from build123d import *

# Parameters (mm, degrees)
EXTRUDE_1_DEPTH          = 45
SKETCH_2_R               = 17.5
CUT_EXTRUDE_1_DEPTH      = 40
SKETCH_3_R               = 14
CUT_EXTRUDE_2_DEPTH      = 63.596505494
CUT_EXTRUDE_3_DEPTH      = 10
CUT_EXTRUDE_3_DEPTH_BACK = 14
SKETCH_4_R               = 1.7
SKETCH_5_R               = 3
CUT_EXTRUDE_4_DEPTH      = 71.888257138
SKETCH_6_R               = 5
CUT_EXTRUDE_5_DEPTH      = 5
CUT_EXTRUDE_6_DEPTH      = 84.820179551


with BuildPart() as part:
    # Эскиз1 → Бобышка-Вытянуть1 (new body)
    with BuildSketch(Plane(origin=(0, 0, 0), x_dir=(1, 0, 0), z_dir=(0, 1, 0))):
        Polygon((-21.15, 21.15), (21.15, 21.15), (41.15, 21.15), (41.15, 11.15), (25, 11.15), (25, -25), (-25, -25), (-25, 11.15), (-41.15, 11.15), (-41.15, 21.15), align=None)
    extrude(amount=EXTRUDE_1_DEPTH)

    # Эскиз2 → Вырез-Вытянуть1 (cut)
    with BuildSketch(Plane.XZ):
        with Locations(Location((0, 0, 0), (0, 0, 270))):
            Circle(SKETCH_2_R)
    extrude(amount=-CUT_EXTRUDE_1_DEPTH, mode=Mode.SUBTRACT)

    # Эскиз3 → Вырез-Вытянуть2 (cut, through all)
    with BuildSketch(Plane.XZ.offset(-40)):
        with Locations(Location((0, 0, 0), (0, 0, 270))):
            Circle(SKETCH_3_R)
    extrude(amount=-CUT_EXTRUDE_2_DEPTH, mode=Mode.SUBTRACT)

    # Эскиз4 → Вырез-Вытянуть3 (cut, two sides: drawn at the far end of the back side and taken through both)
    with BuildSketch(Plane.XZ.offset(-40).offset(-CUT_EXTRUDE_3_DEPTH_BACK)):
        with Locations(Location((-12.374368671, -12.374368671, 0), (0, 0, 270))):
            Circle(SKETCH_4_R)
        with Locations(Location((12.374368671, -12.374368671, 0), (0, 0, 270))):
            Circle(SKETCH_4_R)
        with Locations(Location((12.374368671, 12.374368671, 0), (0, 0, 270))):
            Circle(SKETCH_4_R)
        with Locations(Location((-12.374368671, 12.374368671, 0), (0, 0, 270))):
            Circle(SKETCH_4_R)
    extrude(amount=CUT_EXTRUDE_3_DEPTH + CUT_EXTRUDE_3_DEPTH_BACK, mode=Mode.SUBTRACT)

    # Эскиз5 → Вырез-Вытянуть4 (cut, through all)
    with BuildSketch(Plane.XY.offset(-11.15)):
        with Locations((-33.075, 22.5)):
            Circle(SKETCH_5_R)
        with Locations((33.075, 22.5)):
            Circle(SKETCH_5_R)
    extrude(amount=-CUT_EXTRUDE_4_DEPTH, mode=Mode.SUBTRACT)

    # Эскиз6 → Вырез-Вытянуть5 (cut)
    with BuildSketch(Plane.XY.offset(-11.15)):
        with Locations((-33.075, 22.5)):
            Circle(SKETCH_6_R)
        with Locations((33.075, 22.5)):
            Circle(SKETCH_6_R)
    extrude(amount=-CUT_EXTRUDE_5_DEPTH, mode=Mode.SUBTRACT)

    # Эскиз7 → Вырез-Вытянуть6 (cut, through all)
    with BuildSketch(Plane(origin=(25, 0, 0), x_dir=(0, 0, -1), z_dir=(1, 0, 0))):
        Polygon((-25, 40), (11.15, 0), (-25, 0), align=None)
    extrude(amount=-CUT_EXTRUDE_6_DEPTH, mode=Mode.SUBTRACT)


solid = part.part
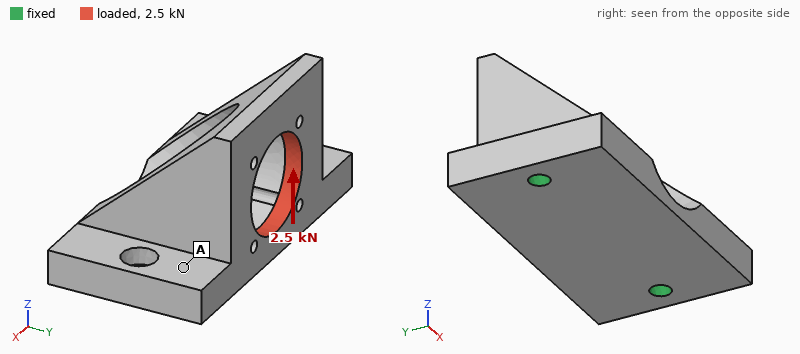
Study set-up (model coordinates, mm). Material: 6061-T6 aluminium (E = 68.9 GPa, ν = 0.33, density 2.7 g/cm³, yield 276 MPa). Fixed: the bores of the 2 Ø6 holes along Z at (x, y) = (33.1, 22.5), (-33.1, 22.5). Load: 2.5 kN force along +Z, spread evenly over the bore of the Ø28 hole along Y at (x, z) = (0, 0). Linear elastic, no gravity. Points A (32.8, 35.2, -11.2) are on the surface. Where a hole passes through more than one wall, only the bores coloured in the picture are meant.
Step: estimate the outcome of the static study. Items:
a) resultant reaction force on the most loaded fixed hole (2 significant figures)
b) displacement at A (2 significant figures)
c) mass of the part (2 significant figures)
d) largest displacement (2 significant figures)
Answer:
1.3 kN
0.042 mm
140 g
0.16 mm
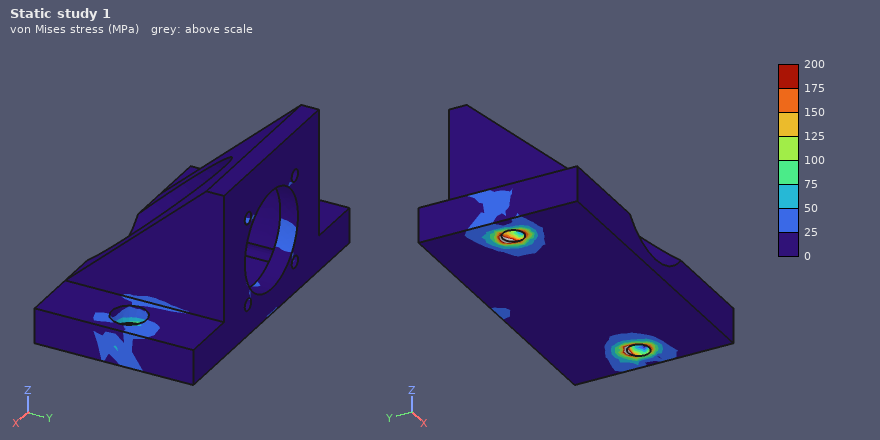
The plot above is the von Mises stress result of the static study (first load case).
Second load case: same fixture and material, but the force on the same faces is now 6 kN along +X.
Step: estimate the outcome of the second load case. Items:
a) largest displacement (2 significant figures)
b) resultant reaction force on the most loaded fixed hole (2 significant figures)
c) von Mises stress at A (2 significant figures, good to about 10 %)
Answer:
58 µm
3.8 kN
16 MPa
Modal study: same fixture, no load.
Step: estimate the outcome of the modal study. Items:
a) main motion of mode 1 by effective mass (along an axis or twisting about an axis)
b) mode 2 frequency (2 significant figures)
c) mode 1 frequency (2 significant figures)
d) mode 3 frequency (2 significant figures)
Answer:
along Y
6300 Hz
2500 Hz
6500 Hz
